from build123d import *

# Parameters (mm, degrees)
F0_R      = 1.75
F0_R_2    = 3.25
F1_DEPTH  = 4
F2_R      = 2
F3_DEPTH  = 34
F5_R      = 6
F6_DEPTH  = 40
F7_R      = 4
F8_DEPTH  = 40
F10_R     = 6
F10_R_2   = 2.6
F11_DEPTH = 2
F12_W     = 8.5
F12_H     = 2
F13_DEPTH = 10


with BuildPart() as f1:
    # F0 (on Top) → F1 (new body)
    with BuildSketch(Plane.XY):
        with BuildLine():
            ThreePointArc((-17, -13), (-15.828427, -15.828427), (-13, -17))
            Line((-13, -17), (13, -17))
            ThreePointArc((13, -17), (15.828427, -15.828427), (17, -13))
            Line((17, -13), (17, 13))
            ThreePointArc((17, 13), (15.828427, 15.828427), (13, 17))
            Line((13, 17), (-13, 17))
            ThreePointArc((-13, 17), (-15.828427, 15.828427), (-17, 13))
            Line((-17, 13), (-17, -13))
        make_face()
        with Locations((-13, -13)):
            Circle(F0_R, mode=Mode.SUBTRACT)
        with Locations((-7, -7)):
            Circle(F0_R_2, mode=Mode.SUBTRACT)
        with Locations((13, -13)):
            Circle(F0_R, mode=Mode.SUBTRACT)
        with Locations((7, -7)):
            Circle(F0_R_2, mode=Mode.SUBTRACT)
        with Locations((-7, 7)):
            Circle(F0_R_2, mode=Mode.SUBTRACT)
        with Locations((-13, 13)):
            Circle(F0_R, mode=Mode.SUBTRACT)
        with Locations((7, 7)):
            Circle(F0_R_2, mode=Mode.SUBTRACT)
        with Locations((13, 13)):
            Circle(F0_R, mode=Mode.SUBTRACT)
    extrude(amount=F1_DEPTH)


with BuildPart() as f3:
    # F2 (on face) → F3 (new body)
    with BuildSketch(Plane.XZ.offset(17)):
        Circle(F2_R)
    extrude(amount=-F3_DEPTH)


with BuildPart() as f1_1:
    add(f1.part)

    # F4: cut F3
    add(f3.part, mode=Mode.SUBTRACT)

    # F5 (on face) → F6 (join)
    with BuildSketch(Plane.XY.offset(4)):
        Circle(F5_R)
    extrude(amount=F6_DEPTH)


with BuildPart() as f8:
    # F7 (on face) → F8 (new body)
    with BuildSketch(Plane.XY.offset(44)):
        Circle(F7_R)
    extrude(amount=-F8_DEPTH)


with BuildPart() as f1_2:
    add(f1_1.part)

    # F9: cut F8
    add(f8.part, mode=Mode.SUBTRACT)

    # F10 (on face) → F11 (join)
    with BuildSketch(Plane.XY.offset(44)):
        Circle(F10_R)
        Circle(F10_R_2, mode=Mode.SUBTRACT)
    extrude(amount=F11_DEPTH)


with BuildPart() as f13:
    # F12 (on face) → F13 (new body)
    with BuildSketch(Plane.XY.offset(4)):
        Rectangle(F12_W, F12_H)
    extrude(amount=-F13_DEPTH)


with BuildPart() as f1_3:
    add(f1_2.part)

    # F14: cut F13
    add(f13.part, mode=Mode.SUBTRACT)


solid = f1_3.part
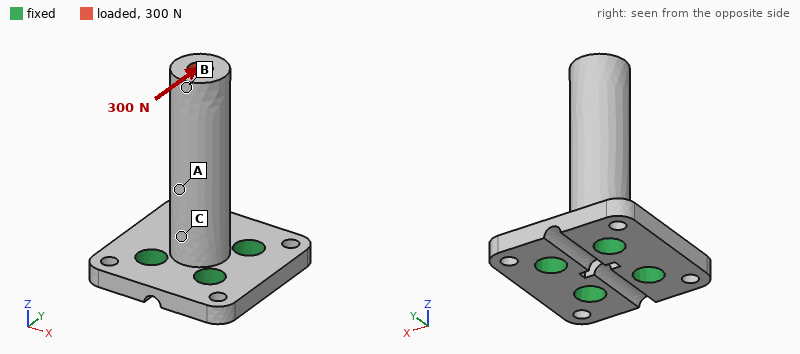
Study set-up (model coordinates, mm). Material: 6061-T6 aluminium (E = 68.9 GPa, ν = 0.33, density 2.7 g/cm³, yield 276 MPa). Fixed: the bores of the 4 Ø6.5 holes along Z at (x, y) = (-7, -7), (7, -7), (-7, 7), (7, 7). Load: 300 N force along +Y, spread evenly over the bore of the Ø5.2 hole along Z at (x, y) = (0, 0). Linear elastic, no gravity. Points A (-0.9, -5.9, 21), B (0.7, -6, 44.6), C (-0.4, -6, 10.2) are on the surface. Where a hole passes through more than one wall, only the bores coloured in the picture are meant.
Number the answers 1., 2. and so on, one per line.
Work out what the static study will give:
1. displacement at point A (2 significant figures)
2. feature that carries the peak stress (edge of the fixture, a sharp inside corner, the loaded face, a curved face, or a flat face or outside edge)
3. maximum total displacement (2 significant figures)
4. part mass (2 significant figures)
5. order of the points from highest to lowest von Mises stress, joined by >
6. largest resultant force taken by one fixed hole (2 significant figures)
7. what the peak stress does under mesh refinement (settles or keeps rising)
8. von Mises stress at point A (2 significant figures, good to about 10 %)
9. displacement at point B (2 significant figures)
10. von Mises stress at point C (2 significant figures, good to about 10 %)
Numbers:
1. 0.049 mm
2. a sharp inside corner
3. 0.17 mm
4. 17 g
5. C > A > B
6. 680 N
7. keeps rising
8. 52 MPa
9. 0.16 mm
10. 74 MPa
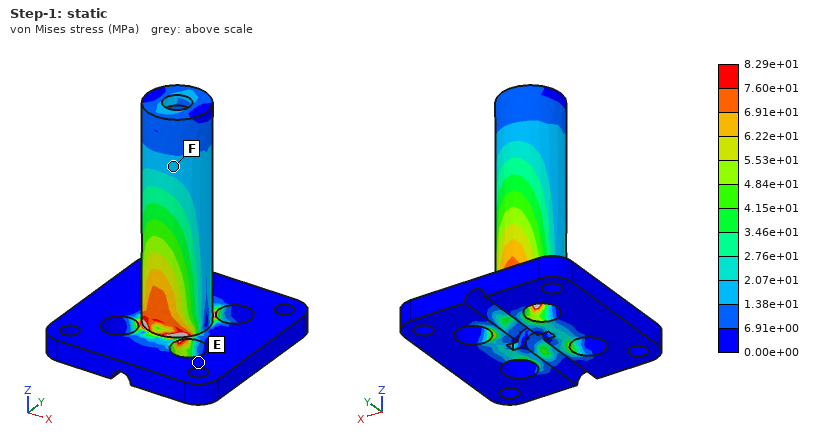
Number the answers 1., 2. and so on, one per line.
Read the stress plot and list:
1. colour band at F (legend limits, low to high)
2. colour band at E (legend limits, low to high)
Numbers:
1. 1.38e+01 to 2.07e+01 MPa
2. 0.00e+00 to 6.91e+00 MPa
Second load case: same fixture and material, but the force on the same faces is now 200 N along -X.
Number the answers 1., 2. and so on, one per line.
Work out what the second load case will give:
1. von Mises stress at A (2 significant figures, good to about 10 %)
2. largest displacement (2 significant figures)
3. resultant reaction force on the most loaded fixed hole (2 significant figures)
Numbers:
1. 11 MPa
2. 0.11 mm
3. 430 N
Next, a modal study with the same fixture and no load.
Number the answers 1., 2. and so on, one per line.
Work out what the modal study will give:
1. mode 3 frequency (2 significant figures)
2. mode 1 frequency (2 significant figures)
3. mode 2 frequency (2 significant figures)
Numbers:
1. 18 kHz
2. 4600 Hz
3. 4600 Hz
